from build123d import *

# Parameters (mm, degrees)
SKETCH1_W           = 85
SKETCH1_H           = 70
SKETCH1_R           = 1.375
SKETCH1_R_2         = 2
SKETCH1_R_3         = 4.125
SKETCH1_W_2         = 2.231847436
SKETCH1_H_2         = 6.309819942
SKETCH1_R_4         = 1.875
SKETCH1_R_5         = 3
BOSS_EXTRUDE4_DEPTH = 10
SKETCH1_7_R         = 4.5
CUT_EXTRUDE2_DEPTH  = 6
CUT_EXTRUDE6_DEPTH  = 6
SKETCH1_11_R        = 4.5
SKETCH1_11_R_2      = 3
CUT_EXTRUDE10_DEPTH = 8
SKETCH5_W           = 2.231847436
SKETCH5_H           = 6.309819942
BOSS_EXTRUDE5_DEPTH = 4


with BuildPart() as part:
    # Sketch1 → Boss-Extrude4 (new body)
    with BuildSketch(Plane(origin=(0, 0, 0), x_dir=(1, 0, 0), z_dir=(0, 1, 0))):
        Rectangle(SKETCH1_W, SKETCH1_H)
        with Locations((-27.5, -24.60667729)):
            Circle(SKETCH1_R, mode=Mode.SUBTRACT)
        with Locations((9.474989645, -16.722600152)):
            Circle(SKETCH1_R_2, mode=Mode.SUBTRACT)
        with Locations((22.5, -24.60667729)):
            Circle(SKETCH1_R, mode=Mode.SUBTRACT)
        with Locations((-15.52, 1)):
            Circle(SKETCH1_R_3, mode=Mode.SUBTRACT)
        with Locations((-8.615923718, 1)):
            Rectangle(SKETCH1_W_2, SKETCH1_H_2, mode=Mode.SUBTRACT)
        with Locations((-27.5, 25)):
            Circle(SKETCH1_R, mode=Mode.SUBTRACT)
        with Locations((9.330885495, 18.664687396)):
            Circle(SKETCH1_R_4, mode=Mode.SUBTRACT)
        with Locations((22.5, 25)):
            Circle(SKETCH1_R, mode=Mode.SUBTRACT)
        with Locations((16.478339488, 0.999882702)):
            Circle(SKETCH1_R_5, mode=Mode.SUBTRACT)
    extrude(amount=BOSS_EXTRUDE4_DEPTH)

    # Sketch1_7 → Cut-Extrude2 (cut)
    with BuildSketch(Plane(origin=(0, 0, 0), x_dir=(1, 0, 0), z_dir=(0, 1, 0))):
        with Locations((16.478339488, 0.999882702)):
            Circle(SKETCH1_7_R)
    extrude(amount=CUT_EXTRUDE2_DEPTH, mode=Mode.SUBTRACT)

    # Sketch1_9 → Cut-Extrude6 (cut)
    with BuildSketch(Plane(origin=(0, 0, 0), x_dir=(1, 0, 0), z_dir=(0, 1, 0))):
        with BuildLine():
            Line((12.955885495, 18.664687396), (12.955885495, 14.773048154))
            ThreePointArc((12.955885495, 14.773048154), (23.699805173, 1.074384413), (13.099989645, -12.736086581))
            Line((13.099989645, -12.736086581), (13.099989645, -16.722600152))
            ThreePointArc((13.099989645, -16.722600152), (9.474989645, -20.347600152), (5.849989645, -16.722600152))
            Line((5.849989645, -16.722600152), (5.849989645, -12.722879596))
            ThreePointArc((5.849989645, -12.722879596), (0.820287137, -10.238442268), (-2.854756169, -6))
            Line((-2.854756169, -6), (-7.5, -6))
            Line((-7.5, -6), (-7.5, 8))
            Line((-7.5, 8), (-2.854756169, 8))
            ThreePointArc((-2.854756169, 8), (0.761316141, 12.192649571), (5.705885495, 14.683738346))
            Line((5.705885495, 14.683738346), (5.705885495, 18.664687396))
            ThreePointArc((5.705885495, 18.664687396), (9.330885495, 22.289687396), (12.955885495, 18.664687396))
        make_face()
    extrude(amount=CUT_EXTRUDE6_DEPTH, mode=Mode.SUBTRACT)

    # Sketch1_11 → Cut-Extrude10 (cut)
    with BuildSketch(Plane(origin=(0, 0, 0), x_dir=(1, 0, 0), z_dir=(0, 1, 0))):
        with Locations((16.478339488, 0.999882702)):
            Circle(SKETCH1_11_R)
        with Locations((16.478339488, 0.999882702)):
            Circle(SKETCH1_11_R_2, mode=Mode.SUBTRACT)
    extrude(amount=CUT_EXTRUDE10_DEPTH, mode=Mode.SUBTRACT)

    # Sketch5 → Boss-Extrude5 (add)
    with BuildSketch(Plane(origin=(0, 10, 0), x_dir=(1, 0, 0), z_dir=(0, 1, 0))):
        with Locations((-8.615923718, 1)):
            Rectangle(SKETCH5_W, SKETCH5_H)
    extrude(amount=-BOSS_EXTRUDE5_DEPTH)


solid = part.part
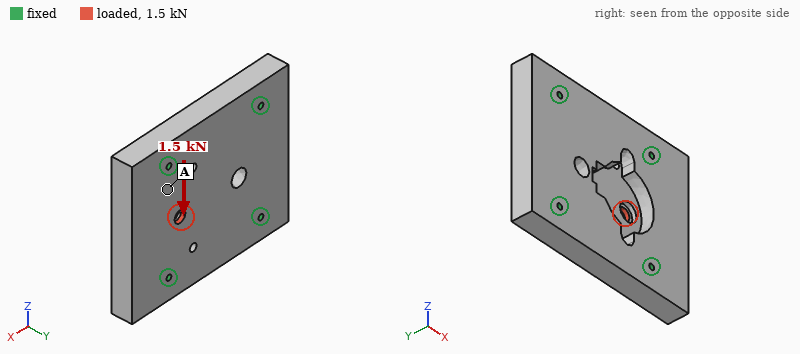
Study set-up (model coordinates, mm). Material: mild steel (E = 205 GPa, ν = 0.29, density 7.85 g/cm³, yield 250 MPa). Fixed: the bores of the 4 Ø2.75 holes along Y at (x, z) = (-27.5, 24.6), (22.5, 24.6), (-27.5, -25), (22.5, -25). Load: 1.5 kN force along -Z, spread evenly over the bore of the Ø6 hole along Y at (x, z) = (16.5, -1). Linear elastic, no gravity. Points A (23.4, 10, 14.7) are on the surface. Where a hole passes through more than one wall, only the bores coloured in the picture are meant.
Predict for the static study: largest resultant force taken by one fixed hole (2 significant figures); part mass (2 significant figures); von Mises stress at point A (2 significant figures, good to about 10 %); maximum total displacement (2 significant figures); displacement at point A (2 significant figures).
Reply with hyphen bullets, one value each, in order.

- 640 N
- 420 g
- 5.5 MPa
- 1.6 µm
- 0.26 µm
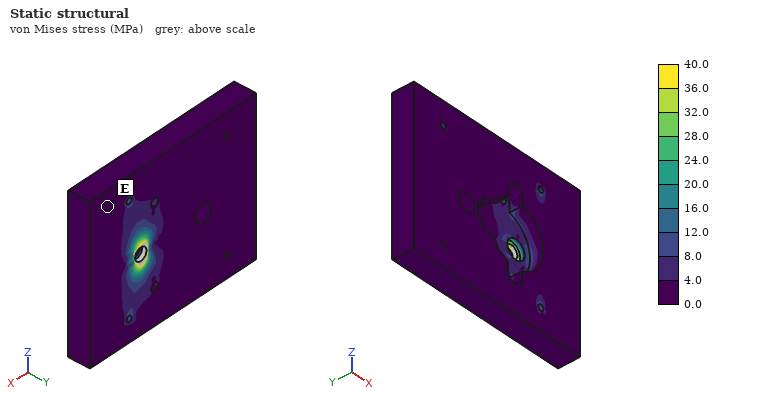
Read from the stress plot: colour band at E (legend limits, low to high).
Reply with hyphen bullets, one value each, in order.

- 0.0 to 4.0 MPa
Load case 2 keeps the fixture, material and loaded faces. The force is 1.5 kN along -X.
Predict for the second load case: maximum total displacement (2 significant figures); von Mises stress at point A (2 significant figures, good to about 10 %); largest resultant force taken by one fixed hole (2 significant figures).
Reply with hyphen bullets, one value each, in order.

- 2.1 µm
- 5.0 MPa
- 480 N
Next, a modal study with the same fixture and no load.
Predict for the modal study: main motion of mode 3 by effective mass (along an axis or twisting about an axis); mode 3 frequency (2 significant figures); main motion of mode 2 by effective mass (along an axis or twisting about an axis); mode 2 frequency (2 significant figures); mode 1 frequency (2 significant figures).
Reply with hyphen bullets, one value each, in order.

- twisting about Z
- 13 kHz
- along Y
- 11 kHz
- 10000 Hz
